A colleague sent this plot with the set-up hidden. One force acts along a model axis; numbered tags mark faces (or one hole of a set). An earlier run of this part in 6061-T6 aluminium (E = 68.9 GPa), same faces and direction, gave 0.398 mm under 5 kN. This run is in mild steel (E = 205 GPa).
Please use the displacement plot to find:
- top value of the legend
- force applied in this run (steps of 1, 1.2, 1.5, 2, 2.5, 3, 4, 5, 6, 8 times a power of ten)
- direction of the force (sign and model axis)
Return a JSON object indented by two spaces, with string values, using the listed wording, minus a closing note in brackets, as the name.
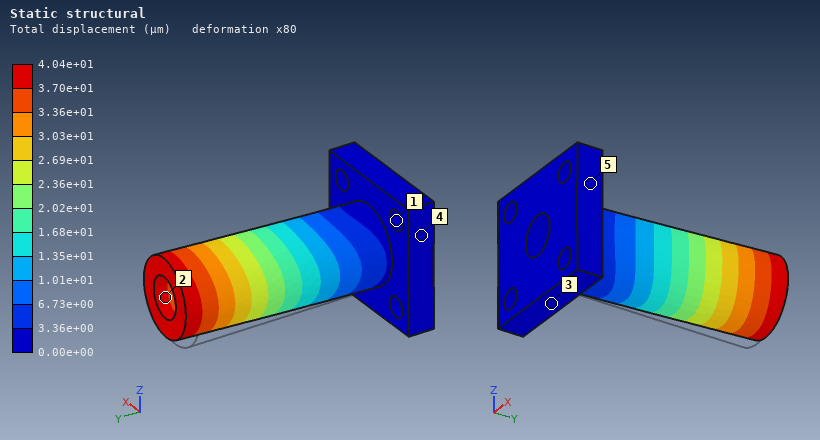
{
  "top value of the legend": "4.04e+01 µm",
  "force applied in this run": "1.5 kN",
  "direction of the force": "+X"
}
